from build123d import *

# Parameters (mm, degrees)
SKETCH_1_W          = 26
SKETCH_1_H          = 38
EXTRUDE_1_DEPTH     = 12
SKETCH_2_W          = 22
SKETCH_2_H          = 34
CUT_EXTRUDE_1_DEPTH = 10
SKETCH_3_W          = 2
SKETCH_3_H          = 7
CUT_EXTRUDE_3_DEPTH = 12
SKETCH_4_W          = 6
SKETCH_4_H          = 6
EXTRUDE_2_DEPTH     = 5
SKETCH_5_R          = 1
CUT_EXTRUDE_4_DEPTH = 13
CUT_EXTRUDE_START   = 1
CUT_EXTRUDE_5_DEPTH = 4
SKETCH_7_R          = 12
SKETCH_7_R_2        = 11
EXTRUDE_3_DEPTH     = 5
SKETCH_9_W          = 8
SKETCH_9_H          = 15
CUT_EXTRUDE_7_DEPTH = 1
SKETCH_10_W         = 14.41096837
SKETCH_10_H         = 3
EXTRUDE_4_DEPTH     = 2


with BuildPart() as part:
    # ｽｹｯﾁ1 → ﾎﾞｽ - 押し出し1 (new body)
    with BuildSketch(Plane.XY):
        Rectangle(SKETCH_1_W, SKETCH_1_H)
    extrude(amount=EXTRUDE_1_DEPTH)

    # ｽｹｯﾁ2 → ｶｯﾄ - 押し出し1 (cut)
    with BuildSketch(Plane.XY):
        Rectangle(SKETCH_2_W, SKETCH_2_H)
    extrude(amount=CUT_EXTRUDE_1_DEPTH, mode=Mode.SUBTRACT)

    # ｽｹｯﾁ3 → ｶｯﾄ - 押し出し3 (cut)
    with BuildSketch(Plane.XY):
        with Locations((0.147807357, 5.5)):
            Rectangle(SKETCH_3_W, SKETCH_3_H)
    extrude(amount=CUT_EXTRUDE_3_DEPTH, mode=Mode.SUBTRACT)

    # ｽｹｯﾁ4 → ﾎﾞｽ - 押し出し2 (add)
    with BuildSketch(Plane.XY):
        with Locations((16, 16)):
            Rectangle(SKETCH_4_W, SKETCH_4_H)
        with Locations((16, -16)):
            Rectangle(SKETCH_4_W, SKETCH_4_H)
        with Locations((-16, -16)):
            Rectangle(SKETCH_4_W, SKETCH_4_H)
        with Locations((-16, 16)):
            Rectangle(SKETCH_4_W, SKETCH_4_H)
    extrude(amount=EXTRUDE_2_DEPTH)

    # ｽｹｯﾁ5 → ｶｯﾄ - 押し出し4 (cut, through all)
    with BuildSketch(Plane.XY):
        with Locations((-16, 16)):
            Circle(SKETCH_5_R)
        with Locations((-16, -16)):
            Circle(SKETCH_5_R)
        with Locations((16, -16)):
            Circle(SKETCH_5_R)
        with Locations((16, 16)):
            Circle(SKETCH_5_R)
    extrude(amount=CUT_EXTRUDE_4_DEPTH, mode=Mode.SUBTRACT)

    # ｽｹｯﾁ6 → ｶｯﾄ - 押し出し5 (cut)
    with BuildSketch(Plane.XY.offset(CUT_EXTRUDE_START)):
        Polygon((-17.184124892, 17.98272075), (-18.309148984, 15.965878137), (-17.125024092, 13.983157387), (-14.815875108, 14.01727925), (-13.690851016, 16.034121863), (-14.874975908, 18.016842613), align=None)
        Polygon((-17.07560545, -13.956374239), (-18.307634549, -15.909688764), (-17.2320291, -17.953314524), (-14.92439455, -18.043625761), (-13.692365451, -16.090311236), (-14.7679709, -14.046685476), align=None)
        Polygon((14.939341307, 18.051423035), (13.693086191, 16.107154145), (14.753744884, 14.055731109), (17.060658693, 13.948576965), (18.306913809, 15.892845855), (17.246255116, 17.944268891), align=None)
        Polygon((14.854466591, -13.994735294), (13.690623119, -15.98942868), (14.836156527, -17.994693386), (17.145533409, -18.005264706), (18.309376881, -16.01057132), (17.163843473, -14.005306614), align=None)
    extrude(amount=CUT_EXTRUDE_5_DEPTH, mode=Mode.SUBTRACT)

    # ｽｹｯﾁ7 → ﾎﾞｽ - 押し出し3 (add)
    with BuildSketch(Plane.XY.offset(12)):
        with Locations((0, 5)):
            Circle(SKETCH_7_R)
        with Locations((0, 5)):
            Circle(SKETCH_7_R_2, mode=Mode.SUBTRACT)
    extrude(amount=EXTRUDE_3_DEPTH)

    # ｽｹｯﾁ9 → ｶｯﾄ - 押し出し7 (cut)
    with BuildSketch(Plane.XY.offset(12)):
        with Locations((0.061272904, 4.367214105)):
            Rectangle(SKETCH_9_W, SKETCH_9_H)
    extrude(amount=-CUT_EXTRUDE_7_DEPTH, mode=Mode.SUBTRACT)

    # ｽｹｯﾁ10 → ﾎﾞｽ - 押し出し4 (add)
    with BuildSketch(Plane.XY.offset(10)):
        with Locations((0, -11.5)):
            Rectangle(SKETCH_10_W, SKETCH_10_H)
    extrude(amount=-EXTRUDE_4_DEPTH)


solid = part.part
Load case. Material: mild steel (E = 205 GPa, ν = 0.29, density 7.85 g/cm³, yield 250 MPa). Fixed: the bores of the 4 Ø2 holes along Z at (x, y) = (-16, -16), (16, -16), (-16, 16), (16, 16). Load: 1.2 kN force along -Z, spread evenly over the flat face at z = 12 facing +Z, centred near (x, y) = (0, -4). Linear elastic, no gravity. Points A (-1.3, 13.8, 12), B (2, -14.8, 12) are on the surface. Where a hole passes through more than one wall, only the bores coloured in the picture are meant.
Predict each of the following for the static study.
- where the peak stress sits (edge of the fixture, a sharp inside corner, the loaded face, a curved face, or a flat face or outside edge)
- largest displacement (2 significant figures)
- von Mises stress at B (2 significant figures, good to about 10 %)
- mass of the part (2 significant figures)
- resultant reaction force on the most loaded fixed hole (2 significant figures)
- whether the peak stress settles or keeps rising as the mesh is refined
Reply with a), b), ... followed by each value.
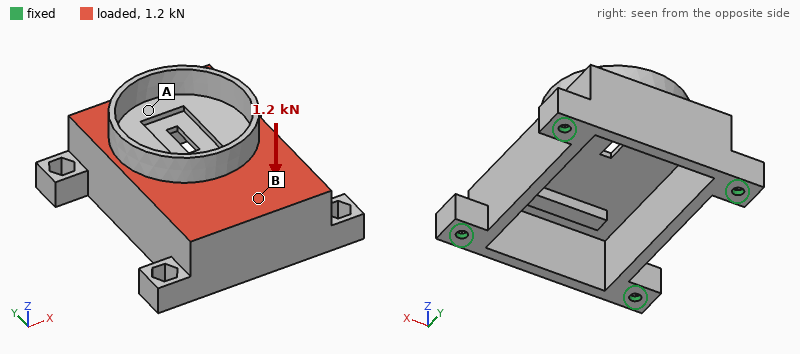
a) edge of the fixture
b) 9.1 µm
c) 19 MPa
d) 41 g
e) 450 N
f) keeps rising
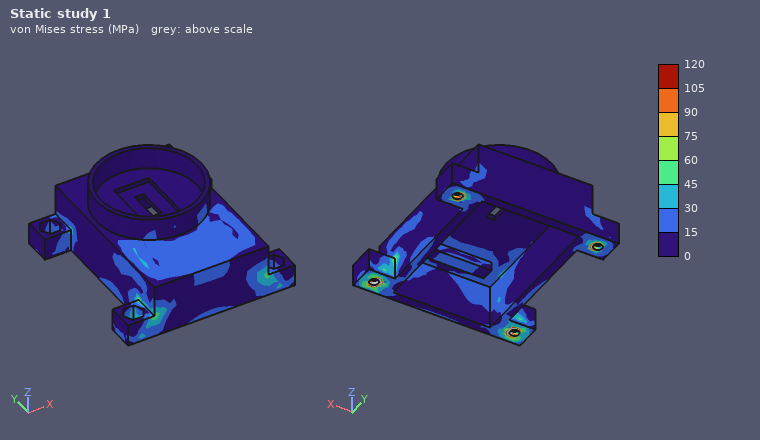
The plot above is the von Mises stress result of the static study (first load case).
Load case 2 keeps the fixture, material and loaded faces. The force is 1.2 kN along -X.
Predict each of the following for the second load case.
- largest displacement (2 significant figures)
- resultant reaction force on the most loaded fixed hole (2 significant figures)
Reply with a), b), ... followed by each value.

a) 5.0 µm
b) 440 N
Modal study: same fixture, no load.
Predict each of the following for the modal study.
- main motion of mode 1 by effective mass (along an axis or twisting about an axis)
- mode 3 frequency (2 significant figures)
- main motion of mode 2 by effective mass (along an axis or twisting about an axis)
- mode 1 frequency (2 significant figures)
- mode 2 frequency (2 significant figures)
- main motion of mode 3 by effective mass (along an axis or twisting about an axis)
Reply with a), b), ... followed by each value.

a) along Y
b) 15 kHz
c) along Z
d) 12 kHz
e) 13 kHz
f) along X
